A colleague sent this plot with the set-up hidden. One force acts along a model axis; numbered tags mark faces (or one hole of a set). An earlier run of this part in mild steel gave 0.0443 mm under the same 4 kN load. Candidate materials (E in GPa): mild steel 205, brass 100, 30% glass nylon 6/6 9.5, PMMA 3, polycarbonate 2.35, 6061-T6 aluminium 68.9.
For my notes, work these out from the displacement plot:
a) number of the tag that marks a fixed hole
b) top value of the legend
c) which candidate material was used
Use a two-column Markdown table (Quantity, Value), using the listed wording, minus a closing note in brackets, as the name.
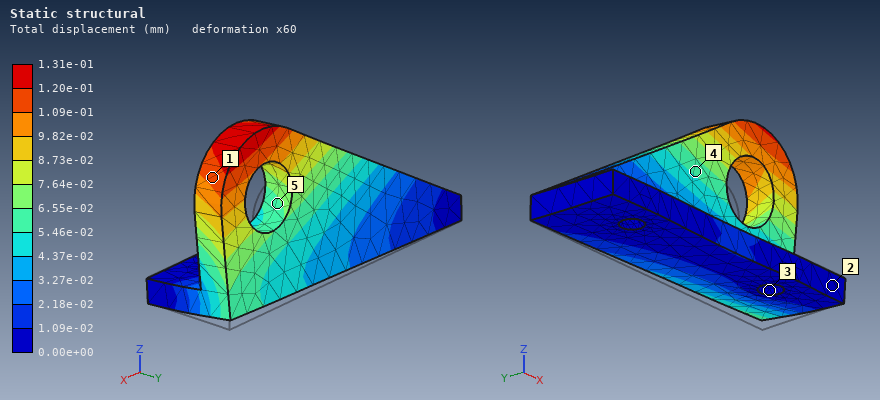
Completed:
| Quantity | Value |
|---|---|
| number of the tag that marks a fixed hole | 3 |
| top value of the legend | 1.31e-01 mm |
| which candidate material was used | 6061-T6 aluminium |
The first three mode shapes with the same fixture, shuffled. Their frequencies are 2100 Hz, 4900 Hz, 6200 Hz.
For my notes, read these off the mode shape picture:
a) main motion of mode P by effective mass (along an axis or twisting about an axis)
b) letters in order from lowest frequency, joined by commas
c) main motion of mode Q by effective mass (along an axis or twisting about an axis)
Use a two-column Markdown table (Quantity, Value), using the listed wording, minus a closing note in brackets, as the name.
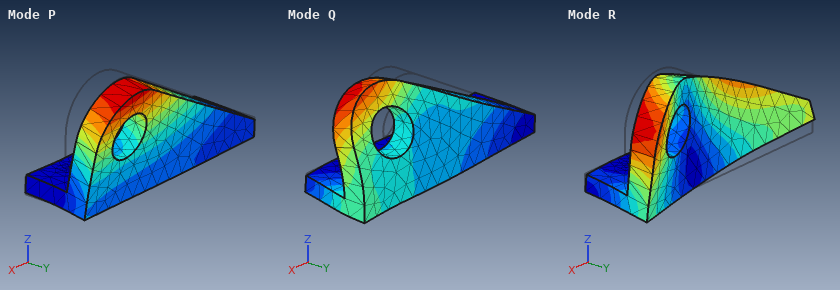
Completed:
| Quantity | Value |
|---|---|
| main motion of mode P by effective mass | along Y |
| letters in order from lowest frequency, joined by commas | P, R, Q |
| main motion of mode Q by effective mass | along Z |
